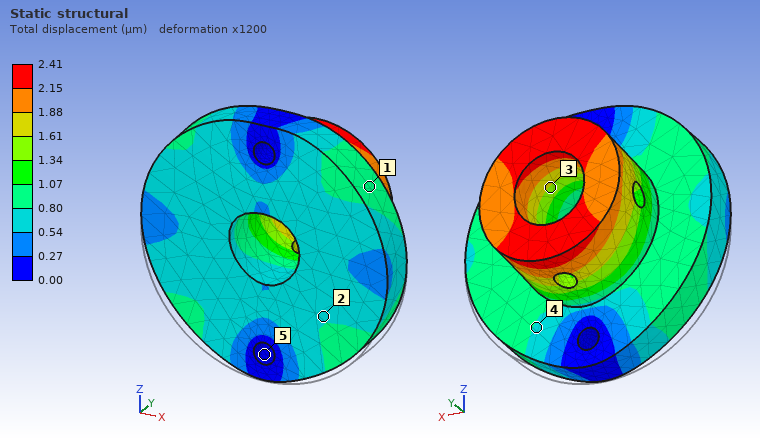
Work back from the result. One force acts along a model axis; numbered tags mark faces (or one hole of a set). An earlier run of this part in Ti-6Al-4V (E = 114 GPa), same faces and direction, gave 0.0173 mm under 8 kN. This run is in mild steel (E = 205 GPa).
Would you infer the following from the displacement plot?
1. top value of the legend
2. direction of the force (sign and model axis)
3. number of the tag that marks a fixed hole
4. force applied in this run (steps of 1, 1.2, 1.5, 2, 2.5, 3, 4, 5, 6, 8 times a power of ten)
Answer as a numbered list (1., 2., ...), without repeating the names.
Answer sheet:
1. 2.41 µm
2. +Z
3. 5
4. 2 kN
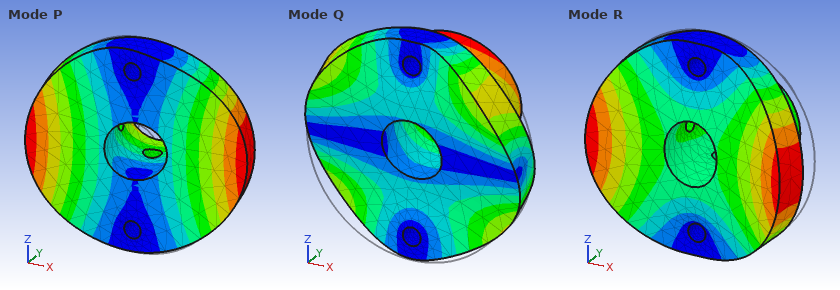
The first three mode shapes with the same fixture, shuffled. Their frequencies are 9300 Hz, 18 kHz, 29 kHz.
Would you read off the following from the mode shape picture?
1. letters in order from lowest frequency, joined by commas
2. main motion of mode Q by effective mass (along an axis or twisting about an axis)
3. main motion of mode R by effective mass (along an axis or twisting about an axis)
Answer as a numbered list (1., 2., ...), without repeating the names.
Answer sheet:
1. P, R, Q
2. along Z
3. along Y
